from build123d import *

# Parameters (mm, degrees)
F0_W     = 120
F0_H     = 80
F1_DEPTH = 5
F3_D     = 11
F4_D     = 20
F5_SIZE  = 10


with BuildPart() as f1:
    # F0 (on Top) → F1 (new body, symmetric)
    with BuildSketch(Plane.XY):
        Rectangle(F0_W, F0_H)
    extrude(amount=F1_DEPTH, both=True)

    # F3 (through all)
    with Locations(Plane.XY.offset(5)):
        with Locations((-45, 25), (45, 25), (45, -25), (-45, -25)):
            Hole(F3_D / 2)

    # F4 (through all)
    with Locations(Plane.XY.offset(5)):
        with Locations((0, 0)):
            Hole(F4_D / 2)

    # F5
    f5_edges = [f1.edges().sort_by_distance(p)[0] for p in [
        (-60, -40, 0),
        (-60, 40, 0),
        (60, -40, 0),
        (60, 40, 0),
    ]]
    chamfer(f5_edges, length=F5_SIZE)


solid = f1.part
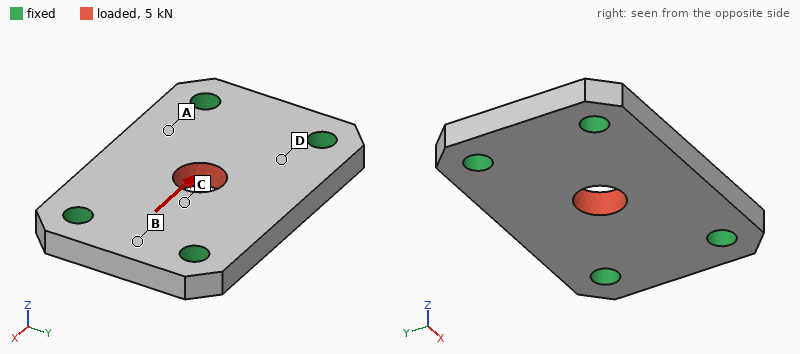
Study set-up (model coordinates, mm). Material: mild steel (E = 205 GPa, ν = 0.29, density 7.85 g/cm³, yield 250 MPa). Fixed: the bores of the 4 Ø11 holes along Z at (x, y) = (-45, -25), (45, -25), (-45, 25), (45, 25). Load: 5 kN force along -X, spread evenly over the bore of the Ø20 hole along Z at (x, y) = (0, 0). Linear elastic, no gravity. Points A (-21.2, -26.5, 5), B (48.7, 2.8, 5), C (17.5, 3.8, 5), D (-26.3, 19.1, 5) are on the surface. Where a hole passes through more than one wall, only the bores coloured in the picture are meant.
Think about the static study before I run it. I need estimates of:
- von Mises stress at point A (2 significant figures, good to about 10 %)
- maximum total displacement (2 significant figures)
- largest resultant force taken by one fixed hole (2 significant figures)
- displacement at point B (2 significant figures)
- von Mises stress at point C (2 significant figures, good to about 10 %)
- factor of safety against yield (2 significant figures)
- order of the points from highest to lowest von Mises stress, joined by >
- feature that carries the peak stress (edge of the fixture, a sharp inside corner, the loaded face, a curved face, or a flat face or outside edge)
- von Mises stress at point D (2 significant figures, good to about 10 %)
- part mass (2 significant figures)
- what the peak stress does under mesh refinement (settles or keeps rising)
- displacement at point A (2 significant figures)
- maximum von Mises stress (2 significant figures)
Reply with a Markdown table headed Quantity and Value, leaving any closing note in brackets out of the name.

| Quantity | Value |
|---|---|
| von Mises stress at point A | 2.9 MPa |
| maximum total displacement | 1.2 µm |
| largest resultant force taken by one fixed hole | 1.3 kN |
| displacement at point B | 0.38 µm |
| von Mises stress at point C | 6.7 MPa |
| factor of safety against yield | 18 |
| order of the points from highest to lowest von Mises stress, joined by > | C > D > A > B |
| feature that carries the peak stress | the loaded face |
| von Mises stress at point D | 5.0 MPa |
| part mass | 680 g |
| what the peak stress does under mesh refinement | settles |
| displacement at point A | 0.37 µm |
| maximum von Mises stress | 14 MPa |
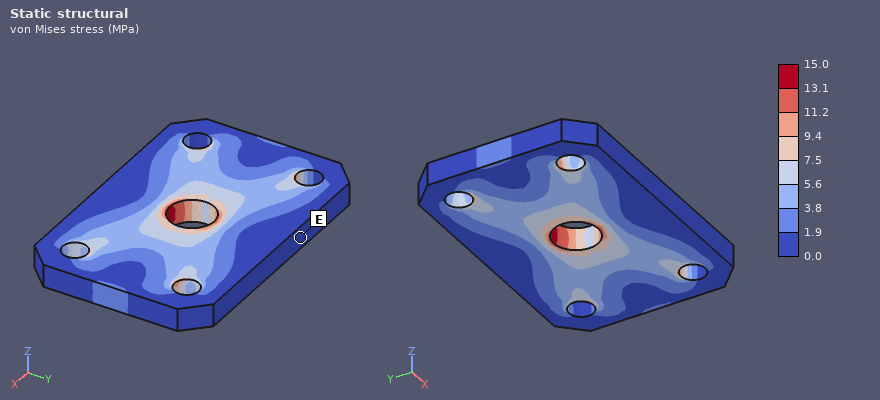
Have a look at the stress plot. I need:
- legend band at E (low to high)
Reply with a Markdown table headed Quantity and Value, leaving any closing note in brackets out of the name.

| Quantity | Value |
|---|---|
| legend band at E | 0.0 to 1.9 MPa |
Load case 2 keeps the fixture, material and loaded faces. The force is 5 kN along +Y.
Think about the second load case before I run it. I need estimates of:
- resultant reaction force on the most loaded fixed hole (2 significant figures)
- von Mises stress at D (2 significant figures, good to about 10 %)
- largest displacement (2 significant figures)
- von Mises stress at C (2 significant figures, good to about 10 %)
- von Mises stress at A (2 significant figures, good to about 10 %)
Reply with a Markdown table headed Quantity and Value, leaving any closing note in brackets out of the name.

| Quantity | Value |
|---|---|
| resultant reaction force on the most loaded fixed hole | 1.5 kN |
| von Mises stress at D | 6.7 MPa |
| largest displacement | 2.2 µm |
| von Mises stress at C | 8.1 MPa |
| von Mises stress at A | 5.0 MPa |
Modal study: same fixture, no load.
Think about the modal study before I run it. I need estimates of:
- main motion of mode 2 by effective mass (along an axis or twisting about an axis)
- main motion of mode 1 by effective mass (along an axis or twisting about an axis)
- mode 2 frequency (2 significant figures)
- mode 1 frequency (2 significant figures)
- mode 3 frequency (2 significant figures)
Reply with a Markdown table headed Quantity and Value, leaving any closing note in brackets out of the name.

| Quantity | Value |
|---|---|
| main motion of mode 2 by effective mass | twisting about X |
| main motion of mode 1 by effective mass | along Z |
| mode 2 frequency | 7900 Hz |
| mode 1 frequency | 6400 Hz |
| mode 3 frequency | 12 kHz |
